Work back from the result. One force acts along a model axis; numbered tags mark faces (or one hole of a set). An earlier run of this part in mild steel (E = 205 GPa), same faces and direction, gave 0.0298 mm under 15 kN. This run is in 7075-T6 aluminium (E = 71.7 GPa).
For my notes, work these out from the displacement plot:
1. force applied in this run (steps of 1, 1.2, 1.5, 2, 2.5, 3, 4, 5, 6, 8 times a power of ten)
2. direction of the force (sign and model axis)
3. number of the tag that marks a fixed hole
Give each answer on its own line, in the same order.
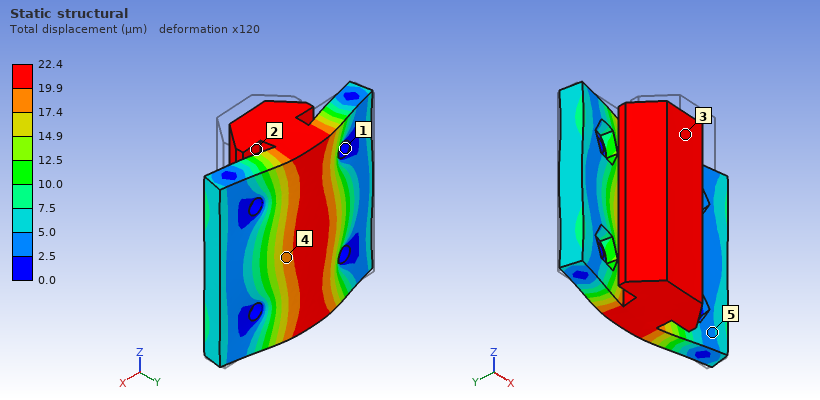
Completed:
4 kN
+Y
1
